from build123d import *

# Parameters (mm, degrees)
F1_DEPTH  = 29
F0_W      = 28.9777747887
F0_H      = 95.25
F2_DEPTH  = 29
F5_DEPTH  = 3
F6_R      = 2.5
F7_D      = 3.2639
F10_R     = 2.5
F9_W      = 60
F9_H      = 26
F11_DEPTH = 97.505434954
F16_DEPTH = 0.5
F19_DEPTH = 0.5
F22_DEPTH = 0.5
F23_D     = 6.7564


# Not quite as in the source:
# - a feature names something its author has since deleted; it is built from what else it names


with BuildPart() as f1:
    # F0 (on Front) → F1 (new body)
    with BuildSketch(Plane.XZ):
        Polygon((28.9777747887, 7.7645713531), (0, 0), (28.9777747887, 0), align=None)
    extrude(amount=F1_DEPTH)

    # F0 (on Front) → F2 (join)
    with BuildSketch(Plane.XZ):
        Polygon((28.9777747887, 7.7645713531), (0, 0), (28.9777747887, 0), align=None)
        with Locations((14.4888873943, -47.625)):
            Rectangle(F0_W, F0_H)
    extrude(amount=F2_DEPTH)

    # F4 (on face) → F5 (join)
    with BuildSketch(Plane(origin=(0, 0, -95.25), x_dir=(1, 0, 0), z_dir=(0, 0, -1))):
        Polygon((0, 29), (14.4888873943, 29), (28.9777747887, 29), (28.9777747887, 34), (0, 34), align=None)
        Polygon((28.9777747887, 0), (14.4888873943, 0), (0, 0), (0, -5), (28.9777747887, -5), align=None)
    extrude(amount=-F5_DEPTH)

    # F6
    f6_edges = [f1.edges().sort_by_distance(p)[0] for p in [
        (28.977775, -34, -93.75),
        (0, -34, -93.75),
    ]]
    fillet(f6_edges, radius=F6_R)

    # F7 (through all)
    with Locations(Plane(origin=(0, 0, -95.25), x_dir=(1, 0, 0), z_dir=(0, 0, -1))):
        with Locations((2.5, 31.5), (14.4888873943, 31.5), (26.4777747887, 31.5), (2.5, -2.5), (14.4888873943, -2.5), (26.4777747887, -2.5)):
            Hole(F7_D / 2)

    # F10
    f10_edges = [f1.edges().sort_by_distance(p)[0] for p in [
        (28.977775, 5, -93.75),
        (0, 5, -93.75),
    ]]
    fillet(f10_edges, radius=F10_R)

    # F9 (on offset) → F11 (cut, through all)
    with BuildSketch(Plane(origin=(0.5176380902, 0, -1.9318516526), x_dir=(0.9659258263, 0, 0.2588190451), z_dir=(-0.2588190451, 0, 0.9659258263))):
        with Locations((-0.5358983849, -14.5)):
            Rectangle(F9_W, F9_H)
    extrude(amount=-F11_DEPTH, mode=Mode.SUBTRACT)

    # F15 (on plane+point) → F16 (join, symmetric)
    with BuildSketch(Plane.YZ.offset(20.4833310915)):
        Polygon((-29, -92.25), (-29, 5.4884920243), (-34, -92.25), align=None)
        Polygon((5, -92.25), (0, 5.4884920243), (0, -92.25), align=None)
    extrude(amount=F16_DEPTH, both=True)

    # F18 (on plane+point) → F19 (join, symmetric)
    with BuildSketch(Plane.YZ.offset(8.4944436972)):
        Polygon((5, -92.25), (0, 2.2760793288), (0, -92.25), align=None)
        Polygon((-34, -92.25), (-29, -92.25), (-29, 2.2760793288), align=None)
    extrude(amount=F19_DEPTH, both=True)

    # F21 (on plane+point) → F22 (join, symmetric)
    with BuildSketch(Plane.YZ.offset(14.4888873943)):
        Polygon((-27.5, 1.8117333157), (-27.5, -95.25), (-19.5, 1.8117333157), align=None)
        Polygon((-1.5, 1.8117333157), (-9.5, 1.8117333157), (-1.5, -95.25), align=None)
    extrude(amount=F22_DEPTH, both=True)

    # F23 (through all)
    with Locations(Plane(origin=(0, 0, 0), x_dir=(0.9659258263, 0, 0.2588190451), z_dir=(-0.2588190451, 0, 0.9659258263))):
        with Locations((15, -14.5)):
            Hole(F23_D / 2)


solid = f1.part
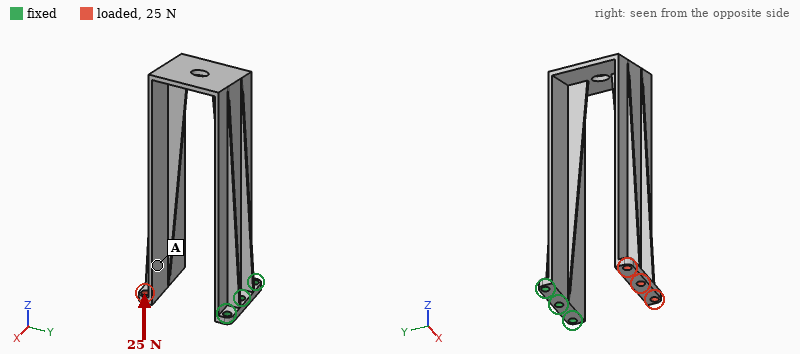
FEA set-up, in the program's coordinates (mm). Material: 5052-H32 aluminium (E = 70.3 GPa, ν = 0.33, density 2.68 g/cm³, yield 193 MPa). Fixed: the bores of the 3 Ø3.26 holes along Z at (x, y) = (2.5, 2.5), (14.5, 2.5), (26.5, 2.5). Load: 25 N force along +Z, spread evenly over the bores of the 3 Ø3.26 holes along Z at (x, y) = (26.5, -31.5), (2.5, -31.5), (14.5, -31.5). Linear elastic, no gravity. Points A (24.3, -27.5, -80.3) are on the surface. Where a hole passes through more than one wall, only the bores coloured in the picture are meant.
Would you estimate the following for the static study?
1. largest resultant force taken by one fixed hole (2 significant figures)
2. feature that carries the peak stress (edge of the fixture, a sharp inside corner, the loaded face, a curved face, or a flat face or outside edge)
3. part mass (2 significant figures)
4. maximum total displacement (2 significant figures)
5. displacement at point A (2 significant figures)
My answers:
19 N
a flat face or outside edge
34 g
1.3 mm
1.0 mm
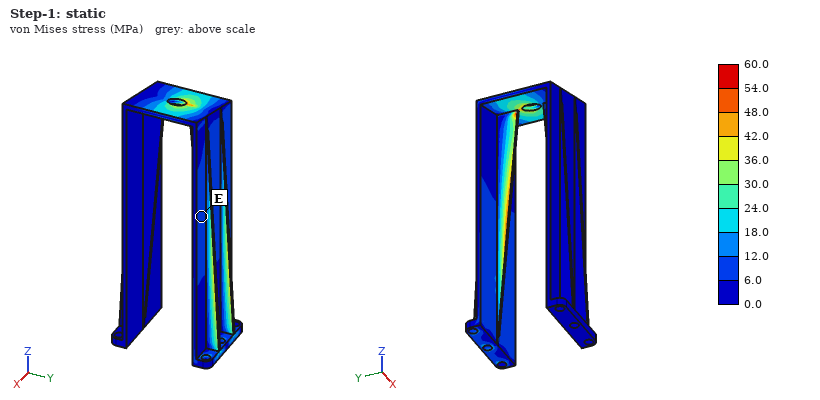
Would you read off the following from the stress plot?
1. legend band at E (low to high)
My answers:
6.0 to 12.0 MPa
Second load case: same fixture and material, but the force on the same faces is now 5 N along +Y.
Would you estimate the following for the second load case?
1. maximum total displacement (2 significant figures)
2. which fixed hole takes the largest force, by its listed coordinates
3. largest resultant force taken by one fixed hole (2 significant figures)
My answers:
1.1 mm
(14.5, 2.5)
2.7 N
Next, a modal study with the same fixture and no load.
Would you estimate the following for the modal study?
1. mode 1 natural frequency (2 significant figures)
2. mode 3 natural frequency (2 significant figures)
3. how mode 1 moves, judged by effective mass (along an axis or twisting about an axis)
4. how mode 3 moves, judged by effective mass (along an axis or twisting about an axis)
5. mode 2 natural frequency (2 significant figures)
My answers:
120 Hz
190 Hz
along X
along Y
150 Hz
